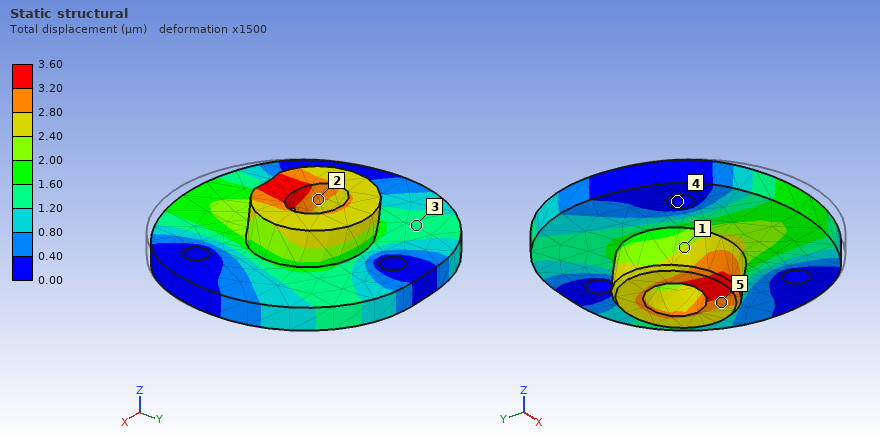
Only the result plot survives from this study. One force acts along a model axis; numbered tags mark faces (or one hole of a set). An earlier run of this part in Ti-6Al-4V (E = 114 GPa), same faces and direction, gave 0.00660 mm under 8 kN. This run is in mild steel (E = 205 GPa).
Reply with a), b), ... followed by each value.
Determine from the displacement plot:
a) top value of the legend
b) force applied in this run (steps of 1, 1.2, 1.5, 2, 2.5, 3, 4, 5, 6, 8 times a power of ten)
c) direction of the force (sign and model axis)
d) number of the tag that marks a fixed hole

a) 3.60 µm
b) 8 kN
c) +Y
d) 4
